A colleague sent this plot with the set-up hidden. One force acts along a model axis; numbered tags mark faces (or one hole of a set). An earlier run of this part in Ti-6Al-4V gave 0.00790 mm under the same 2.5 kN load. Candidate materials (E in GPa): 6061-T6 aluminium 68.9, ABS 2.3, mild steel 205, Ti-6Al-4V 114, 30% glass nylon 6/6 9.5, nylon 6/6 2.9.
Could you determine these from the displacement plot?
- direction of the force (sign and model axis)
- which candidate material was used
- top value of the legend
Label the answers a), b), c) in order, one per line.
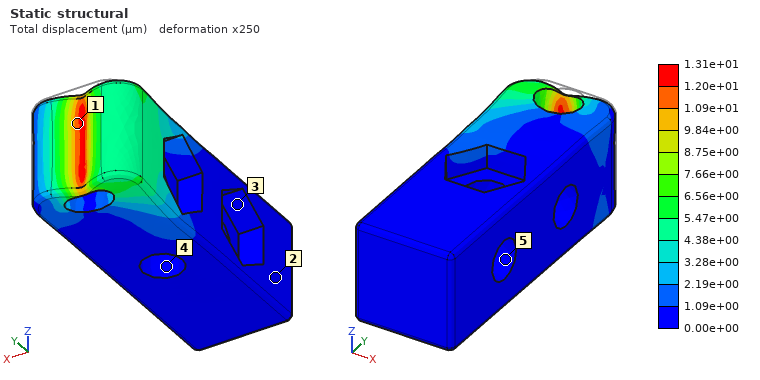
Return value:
a) -Y
b) 6061-T6 aluminium
c) 1.31e+01 µm
